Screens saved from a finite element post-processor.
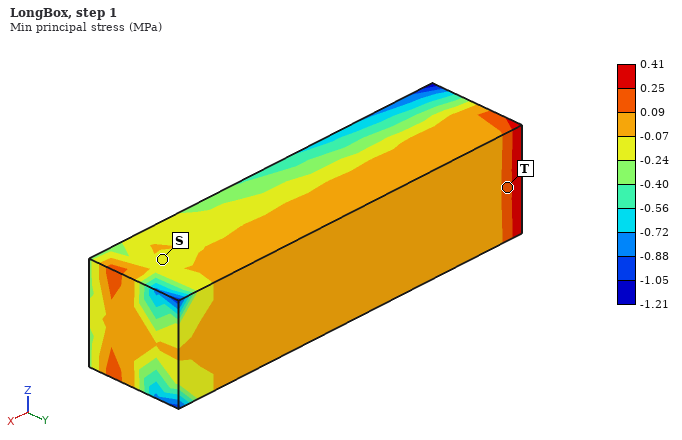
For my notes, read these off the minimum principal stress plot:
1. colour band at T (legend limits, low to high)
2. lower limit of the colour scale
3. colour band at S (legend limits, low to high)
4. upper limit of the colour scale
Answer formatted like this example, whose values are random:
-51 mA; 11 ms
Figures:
0.09 to 0.25 MPa; -1.21 MPa; -0.24 to -0.07 MPa; 0.41 MPa
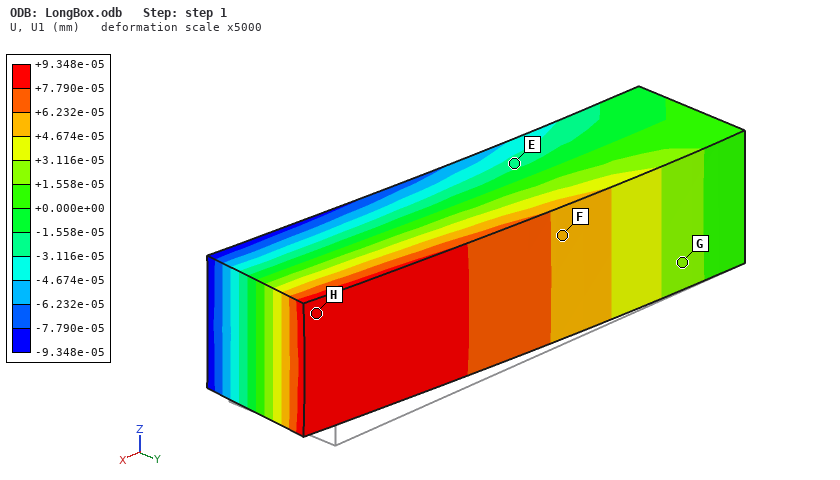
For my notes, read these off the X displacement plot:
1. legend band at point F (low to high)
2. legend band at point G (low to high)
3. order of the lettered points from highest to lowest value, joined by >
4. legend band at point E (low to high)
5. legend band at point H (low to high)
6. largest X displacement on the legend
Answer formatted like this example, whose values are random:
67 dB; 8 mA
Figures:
+4.674e-05 to +6.232e-05 mm; +1.558e-05 to +3.116e-05 mm; H > F > G > E; -3.116e-05 to -1.558e-05 mm; +7.790e-05 to +9.348e-05 mm; +9.348e-05 mm
